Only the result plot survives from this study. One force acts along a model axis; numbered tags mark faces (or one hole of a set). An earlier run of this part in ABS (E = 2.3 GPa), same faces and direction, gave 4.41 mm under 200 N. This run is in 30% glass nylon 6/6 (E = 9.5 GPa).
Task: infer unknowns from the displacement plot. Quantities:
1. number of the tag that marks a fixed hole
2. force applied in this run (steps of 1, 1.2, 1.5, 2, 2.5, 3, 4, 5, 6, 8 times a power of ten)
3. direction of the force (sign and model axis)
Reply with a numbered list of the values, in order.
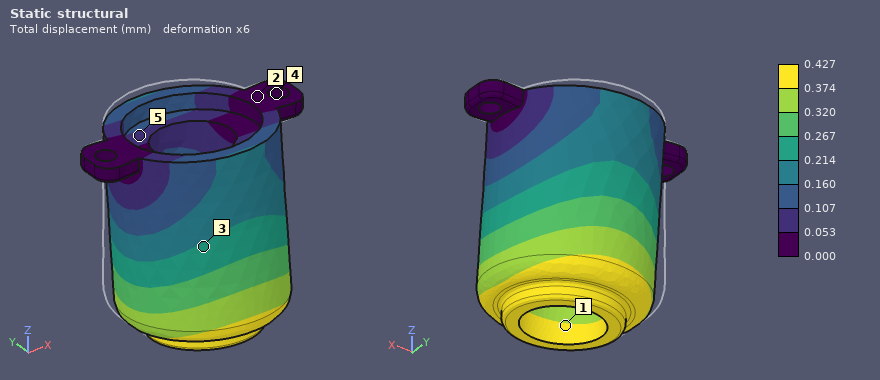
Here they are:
1. 4
2. 80 N
3. -Y
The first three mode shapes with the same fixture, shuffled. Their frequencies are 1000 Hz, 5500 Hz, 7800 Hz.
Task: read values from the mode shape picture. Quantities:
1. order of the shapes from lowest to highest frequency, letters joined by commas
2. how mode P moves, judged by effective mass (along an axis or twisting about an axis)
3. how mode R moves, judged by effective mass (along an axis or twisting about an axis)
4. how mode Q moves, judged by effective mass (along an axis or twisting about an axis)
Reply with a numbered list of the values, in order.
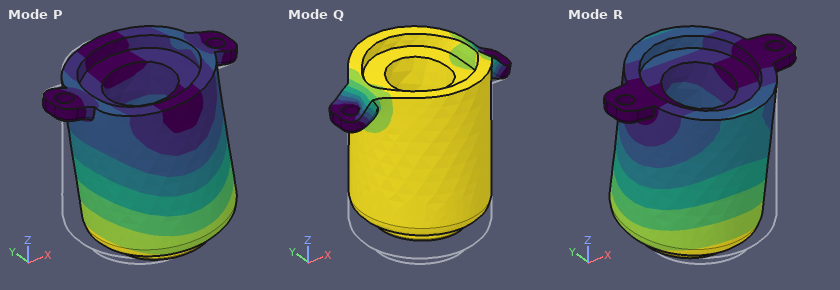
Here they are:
1. R, P, Q
2. along X
3. along Y
4. along Z
